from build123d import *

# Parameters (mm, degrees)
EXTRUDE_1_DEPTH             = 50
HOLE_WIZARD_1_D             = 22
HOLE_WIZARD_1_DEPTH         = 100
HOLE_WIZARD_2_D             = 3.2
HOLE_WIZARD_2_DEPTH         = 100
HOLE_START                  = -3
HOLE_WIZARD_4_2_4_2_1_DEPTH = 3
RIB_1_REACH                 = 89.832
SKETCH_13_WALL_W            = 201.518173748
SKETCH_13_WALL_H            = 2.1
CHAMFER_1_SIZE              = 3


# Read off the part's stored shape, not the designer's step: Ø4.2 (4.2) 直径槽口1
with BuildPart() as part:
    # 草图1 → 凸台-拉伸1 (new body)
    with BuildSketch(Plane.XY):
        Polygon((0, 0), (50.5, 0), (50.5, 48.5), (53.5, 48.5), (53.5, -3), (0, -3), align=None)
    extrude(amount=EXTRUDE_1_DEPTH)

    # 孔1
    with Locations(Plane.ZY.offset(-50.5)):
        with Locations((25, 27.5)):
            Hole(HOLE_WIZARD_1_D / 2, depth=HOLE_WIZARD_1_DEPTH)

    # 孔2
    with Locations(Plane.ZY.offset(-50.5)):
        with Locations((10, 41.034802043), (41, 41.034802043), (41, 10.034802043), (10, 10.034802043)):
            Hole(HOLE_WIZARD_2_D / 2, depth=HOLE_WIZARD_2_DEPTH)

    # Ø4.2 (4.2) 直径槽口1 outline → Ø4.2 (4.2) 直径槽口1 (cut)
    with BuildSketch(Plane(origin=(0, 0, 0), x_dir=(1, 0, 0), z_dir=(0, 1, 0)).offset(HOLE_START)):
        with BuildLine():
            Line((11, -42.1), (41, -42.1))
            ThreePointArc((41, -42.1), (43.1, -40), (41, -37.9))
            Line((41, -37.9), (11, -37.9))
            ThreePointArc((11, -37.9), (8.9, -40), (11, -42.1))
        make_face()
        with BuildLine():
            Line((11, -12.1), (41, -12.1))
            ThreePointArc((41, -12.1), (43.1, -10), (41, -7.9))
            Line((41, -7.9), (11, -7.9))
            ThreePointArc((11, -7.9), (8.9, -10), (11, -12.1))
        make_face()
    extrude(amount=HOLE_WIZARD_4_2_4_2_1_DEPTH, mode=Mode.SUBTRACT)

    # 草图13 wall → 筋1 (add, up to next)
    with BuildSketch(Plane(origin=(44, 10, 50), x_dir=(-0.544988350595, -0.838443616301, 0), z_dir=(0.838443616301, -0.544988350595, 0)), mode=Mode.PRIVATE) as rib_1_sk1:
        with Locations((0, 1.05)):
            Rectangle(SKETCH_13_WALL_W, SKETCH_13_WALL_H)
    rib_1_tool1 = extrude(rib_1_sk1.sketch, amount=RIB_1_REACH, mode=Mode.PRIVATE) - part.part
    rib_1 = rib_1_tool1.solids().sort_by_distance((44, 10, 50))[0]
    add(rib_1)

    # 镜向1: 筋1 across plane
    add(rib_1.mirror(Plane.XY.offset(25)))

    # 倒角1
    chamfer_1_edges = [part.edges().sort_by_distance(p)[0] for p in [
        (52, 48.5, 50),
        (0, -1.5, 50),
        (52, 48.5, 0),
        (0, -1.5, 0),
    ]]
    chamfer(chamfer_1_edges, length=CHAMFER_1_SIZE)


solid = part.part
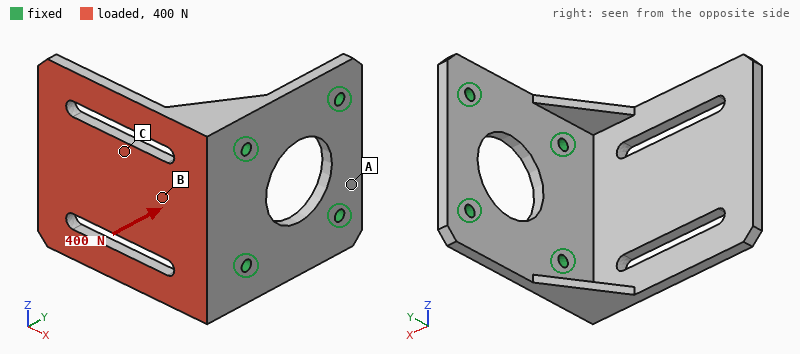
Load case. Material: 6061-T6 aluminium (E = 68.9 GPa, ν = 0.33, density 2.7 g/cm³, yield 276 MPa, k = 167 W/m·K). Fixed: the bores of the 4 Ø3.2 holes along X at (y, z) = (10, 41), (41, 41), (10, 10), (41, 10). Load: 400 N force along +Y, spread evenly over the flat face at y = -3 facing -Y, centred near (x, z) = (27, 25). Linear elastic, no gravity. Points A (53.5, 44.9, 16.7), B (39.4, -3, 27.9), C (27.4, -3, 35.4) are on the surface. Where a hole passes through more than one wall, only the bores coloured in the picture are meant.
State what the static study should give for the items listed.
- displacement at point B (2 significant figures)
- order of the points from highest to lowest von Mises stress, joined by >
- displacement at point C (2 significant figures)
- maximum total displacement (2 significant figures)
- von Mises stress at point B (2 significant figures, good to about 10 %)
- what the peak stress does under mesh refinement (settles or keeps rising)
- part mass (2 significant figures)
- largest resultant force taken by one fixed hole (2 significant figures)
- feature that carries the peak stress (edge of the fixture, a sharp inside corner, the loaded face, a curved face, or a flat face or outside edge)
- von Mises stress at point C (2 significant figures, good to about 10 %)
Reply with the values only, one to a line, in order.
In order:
0.16 mm
B > C > A
0.35 mm
0.98 mm
54 MPa
keeps rising
37 g
210 N
edge of the fixture
31 MPa
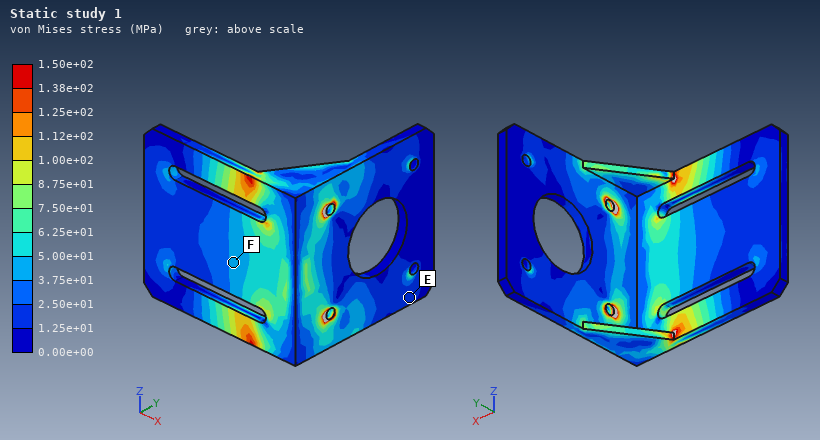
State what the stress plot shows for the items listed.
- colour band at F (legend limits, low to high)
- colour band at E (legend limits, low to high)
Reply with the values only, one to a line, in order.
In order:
3.75e+01 to 5.00e+01 MPa
1.25e+01 to 2.50e+01 MPa
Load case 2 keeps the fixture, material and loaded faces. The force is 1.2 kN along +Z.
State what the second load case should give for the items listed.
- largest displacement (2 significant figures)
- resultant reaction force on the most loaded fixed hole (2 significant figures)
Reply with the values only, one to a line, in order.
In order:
0.29 mm
1.2 kN
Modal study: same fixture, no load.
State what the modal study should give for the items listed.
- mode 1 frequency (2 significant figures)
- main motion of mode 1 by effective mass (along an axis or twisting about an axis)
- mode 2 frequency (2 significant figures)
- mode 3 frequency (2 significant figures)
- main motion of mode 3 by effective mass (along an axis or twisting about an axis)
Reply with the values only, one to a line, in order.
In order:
910 Hz
along Y
2200 Hz
3200 Hz
along Z
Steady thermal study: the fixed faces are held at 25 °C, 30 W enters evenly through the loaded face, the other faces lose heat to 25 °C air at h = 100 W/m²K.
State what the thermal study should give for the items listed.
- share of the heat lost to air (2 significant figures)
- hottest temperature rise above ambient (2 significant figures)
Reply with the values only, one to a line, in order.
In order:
32 %
32 K
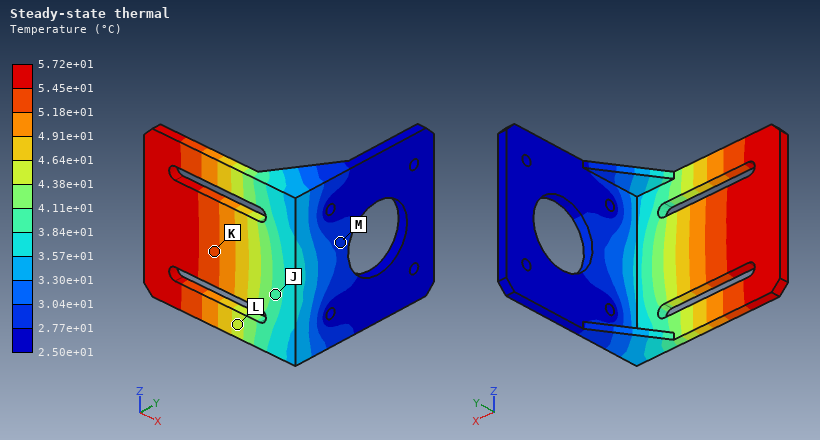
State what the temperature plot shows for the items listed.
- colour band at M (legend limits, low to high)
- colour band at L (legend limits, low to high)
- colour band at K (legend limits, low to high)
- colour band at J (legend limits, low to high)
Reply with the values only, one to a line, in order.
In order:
2.77e+01 to 3.04e+01 °C
4.38e+01 to 4.64e+01 °C
5.18e+01 to 5.45e+01 °C
3.84e+01 to 4.11e+01 °C
